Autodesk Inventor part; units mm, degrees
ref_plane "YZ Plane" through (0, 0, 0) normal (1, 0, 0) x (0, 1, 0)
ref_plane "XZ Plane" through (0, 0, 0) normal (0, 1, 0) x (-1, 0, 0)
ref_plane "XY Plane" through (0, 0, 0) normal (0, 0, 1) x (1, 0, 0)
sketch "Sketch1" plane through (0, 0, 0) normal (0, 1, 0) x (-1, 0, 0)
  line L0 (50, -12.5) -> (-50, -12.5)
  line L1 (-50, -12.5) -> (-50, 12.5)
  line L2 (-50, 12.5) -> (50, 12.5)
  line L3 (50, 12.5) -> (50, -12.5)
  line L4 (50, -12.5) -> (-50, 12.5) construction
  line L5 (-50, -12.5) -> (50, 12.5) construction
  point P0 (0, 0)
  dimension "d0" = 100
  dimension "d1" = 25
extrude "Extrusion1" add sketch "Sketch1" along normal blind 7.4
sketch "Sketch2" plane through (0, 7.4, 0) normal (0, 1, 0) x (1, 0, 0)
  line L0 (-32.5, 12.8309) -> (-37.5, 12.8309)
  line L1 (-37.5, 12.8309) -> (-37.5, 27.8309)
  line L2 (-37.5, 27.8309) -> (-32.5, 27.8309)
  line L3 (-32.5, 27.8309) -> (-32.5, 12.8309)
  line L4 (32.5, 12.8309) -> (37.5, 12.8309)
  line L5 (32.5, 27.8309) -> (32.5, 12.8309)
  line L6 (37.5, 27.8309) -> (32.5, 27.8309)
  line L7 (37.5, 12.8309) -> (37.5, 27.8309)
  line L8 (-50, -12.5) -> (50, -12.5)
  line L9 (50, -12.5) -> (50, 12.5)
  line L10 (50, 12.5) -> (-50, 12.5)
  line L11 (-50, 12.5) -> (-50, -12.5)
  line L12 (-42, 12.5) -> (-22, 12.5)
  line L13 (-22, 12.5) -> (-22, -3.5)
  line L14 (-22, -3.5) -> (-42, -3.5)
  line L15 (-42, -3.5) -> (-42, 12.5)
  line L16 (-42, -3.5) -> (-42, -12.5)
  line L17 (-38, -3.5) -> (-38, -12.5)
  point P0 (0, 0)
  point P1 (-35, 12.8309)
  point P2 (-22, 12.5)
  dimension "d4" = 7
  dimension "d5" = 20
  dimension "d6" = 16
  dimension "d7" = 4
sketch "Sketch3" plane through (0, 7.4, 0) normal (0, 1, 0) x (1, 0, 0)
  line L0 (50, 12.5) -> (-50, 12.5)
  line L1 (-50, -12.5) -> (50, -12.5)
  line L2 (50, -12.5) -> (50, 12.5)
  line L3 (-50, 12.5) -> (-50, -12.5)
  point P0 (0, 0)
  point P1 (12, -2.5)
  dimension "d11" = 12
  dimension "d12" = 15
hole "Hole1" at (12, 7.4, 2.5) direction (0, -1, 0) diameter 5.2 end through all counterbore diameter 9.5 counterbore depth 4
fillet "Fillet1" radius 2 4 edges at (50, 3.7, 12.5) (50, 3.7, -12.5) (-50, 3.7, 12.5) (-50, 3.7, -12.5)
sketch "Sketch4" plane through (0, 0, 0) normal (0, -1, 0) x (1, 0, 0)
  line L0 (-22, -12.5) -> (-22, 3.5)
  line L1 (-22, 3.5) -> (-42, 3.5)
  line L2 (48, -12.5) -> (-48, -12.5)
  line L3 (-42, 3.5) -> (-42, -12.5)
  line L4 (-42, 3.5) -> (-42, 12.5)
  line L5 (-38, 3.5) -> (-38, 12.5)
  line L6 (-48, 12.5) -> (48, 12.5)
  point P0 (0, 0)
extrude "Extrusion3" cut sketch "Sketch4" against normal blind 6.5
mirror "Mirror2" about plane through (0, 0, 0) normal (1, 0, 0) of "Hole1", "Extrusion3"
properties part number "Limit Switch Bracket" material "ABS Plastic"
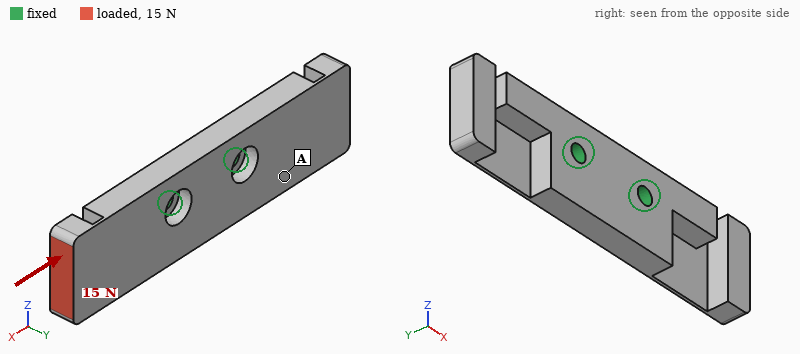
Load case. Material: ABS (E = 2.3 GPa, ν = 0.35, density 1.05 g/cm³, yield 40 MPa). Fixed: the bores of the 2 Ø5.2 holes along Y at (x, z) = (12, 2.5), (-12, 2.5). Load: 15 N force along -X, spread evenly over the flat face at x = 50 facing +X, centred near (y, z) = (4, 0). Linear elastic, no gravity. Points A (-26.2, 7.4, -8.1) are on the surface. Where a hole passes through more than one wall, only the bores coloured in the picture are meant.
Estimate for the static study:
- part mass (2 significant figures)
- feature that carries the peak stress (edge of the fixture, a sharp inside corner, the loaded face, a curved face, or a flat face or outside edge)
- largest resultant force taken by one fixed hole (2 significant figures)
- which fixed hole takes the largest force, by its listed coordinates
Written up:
14 g
a flat face or outside edge
11 N
(12, 2.5)
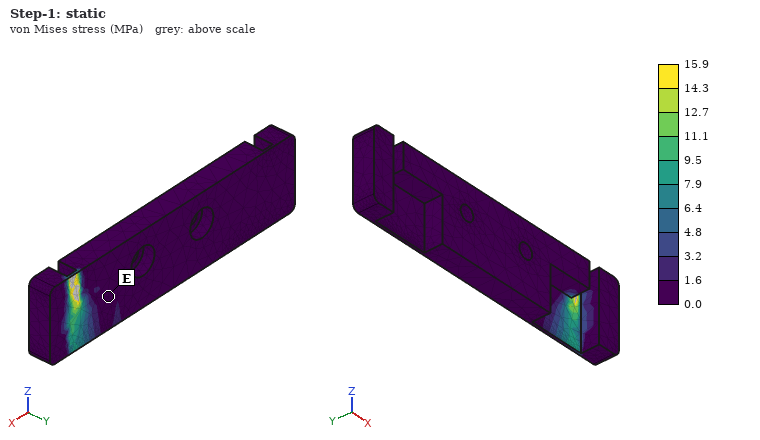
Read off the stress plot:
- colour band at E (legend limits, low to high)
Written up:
0.0 to 1.6 MPa
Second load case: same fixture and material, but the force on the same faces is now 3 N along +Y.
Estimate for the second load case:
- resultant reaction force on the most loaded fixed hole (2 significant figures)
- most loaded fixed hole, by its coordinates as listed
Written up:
8.3 N
(12, 2.5)
